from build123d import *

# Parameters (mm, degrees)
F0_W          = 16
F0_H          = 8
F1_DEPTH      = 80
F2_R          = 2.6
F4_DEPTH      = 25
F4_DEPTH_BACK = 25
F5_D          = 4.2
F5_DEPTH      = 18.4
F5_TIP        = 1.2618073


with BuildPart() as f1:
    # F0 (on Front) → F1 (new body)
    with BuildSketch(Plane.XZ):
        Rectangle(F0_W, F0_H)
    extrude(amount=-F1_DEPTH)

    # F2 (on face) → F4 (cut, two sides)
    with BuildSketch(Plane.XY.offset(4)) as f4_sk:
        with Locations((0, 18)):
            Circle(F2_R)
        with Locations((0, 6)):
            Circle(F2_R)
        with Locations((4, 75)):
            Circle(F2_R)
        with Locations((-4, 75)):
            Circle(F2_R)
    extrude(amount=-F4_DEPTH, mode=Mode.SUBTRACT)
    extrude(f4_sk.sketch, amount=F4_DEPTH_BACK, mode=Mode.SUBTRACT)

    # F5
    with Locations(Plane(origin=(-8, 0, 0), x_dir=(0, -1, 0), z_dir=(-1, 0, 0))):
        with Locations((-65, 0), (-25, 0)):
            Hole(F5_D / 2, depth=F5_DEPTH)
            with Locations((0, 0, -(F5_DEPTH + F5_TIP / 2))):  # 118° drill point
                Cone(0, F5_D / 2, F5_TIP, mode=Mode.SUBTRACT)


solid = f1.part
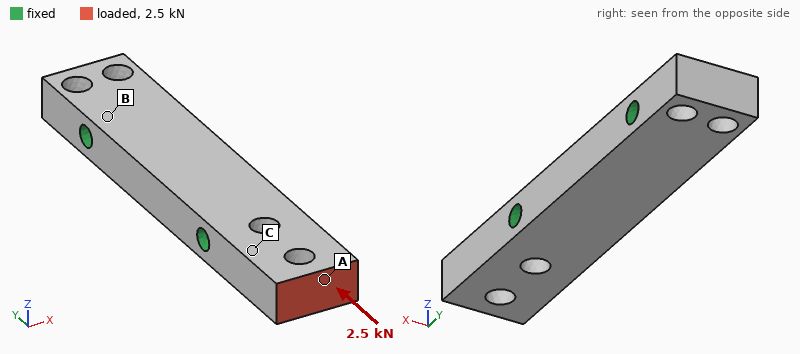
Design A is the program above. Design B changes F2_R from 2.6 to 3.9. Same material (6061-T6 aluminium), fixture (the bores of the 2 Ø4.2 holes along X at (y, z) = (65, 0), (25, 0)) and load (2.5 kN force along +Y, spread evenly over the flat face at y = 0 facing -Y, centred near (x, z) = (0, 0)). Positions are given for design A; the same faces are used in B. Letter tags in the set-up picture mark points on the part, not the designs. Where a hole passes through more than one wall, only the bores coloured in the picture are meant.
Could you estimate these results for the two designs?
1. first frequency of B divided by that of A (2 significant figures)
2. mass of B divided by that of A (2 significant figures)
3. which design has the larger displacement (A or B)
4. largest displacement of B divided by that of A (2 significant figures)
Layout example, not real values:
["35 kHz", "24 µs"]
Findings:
["0.95", "0.91", "B", "1.8"]
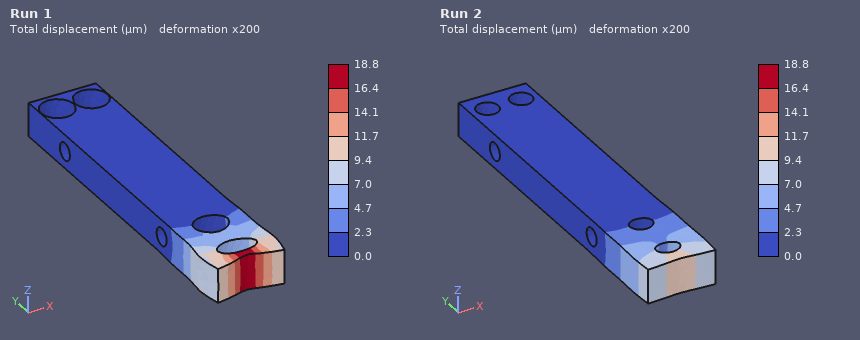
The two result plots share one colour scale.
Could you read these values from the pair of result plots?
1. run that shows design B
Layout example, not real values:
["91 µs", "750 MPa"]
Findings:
["Run 1"]
